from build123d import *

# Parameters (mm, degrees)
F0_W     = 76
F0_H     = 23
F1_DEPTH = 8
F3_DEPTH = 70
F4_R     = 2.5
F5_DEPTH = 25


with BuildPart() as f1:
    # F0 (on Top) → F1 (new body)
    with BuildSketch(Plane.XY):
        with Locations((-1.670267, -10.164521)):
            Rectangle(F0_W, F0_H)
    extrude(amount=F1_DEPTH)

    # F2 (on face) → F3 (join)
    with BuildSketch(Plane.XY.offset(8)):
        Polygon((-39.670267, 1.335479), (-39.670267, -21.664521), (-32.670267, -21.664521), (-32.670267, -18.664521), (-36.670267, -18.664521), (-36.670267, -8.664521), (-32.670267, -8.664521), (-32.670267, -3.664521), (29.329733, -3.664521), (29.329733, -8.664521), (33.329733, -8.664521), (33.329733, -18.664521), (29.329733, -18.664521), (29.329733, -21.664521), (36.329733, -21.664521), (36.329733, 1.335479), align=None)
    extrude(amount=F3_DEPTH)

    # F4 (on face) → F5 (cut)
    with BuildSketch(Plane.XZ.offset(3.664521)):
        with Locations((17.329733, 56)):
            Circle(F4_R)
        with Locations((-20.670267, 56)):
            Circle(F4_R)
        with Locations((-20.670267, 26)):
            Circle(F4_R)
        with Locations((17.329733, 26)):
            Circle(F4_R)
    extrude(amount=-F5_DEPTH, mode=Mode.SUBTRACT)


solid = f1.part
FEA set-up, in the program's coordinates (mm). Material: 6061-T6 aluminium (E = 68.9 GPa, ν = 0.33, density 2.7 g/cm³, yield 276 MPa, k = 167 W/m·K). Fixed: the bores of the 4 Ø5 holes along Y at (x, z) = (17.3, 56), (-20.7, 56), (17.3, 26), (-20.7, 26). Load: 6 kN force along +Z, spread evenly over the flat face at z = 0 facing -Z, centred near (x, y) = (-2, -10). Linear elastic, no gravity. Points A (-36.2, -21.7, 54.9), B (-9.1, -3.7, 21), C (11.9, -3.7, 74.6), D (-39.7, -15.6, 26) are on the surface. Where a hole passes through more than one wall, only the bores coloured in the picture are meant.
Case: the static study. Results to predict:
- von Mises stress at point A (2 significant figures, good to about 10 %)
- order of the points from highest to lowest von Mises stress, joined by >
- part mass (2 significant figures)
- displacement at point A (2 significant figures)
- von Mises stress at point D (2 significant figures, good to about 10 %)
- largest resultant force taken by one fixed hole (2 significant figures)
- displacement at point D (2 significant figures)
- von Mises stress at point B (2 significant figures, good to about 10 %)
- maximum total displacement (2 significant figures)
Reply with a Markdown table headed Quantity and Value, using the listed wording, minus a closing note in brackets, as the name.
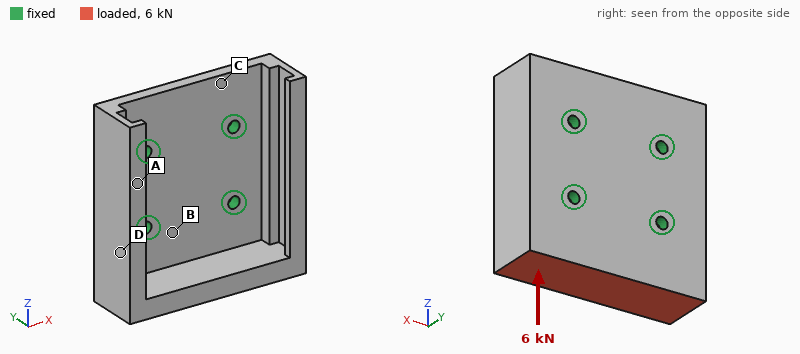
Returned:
| Quantity | Value |
|---|---|
| von Mises stress at point A | 7.4 MPa |
| order of the points from highest to lowest von Mises stress, joined by > | B > D > C > A |
| part mass | 140 g |
| displacement at point A | 0.057 mm |
| von Mises stress at point D | 27 MPa |
| largest resultant force taken by one fixed hole | 2.2 kN |
| displacement at point D | 0.031 mm |
| von Mises stress at point B | 40 MPa |
| maximum total displacement | 0.13 mm |
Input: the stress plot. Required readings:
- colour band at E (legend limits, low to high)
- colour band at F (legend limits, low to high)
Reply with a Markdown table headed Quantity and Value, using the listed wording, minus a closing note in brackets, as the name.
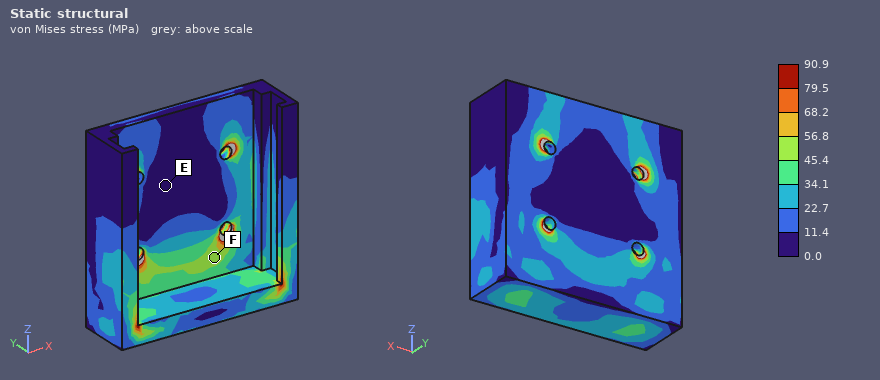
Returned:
| Quantity | Value |
|---|---|
| colour band at E | 0.0 to 11.4 MPa |
| colour band at F | 45.4 to 56.8 MPa |
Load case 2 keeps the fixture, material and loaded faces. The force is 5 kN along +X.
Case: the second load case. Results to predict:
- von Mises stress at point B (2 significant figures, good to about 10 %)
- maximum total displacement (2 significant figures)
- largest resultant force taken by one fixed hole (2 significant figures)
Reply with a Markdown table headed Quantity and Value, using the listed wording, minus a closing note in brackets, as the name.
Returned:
| Quantity | Value |
|---|---|
| von Mises stress at point B | 43 MPa |
| maximum total displacement | 89 µm |
| largest resultant force taken by one fixed hole | 3.5 kN |
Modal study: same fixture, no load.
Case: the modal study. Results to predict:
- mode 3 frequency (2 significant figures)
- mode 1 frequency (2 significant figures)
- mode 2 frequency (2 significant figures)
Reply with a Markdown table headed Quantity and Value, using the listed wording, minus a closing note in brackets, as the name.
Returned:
| Quantity | Value |
|---|---|
| mode 3 frequency | 4600 Hz |
| mode 1 frequency | 3700 Hz |
| mode 2 frequency | 4000 Hz |
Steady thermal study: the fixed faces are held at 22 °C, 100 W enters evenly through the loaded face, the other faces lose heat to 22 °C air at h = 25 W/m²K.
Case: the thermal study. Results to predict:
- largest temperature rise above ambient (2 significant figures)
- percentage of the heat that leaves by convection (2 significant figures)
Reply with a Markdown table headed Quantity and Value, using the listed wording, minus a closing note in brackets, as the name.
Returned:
| Quantity | Value |
|---|---|
| largest temperature rise above ambient | 39 K |
| percentage of the heat that leaves by convection | 6.1 % |
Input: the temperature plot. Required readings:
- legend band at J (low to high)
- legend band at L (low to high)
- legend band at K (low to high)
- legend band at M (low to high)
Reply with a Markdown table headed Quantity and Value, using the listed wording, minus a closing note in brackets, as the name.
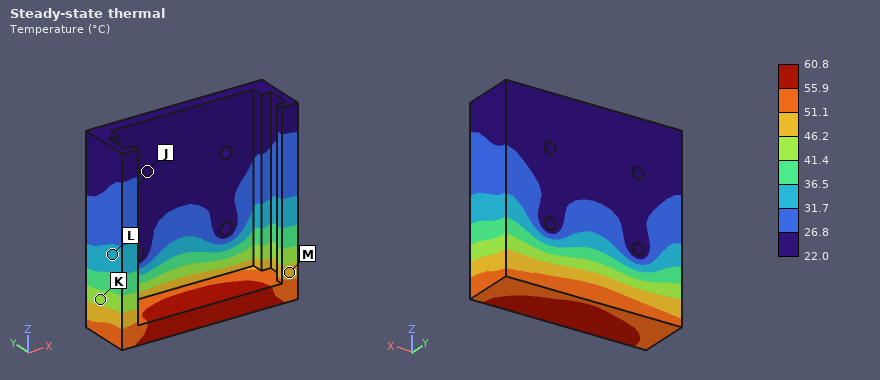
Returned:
| Quantity | Value |
|---|---|
| legend band at J | 22.0 to 26.8 °C |
| legend band at L | 31.7 to 36.5 °C |
| legend band at K | 41.4 to 46.2 °C |
| legend band at M | 46.2 to 51.1 °C |
